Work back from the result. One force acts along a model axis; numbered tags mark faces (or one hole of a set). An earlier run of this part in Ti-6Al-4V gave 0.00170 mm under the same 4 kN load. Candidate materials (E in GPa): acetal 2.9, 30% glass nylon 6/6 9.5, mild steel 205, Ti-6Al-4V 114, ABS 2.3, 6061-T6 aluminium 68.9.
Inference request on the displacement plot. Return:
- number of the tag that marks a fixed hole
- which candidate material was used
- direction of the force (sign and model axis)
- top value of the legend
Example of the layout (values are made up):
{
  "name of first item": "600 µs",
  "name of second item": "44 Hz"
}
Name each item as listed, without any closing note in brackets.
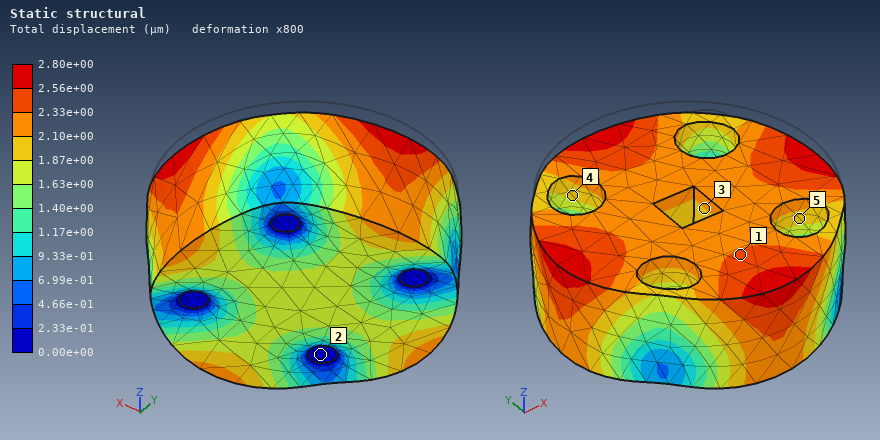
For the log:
{
  "number of the tag that marks a fixed hole": "2",
  "which candidate material was used": "6061-T6 aluminium",
  "direction of the force": "-Z",
  "top value of the legend": "2.80e+00 µm"
}
